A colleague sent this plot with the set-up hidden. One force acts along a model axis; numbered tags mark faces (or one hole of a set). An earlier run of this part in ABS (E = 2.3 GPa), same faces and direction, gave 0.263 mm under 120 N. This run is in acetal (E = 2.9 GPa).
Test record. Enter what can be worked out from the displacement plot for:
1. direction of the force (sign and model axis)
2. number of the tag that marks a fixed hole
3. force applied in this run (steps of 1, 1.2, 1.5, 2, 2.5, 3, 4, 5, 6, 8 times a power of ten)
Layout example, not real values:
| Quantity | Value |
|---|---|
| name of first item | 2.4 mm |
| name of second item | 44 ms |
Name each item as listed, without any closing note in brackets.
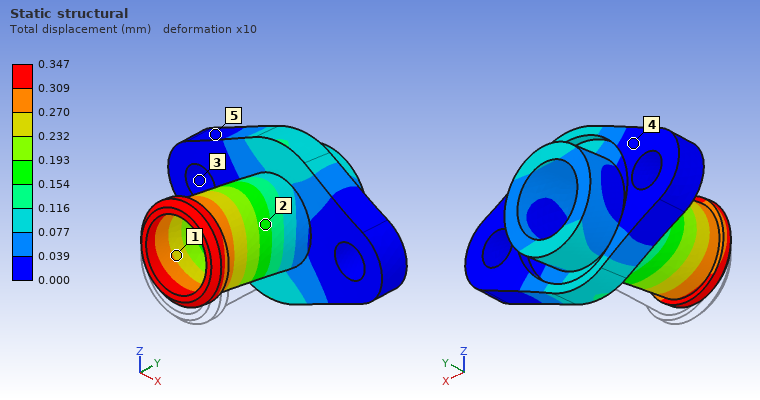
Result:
| Quantity | Value |
|---|---|
| direction of the force | +Z |
| number of the tag that marks a fixed hole | 3 |
| force applied in this run | 200 N |
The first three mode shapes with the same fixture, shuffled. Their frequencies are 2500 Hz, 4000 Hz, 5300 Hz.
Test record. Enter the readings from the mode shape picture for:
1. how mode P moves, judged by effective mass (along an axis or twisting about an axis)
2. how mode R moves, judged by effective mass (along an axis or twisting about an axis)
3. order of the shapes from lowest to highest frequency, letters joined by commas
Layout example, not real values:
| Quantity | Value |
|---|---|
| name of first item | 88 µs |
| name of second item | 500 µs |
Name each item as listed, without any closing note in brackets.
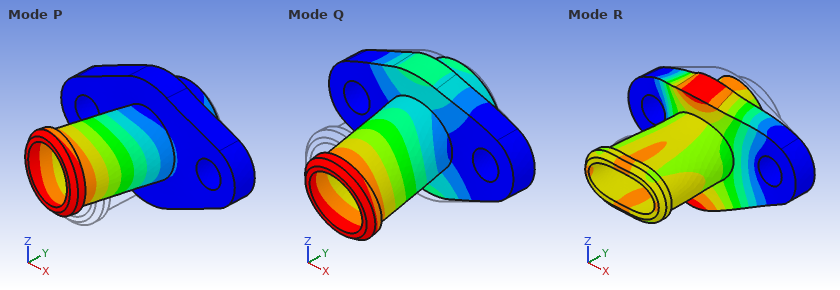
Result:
| Quantity | Value |
|---|---|
| how mode P moves, judged by effective mass | along X |
| how mode R moves, judged by effective mass | along Y |
| order of the shapes from lowest to highest frequency, letters joined by commas | Q, P, R |
